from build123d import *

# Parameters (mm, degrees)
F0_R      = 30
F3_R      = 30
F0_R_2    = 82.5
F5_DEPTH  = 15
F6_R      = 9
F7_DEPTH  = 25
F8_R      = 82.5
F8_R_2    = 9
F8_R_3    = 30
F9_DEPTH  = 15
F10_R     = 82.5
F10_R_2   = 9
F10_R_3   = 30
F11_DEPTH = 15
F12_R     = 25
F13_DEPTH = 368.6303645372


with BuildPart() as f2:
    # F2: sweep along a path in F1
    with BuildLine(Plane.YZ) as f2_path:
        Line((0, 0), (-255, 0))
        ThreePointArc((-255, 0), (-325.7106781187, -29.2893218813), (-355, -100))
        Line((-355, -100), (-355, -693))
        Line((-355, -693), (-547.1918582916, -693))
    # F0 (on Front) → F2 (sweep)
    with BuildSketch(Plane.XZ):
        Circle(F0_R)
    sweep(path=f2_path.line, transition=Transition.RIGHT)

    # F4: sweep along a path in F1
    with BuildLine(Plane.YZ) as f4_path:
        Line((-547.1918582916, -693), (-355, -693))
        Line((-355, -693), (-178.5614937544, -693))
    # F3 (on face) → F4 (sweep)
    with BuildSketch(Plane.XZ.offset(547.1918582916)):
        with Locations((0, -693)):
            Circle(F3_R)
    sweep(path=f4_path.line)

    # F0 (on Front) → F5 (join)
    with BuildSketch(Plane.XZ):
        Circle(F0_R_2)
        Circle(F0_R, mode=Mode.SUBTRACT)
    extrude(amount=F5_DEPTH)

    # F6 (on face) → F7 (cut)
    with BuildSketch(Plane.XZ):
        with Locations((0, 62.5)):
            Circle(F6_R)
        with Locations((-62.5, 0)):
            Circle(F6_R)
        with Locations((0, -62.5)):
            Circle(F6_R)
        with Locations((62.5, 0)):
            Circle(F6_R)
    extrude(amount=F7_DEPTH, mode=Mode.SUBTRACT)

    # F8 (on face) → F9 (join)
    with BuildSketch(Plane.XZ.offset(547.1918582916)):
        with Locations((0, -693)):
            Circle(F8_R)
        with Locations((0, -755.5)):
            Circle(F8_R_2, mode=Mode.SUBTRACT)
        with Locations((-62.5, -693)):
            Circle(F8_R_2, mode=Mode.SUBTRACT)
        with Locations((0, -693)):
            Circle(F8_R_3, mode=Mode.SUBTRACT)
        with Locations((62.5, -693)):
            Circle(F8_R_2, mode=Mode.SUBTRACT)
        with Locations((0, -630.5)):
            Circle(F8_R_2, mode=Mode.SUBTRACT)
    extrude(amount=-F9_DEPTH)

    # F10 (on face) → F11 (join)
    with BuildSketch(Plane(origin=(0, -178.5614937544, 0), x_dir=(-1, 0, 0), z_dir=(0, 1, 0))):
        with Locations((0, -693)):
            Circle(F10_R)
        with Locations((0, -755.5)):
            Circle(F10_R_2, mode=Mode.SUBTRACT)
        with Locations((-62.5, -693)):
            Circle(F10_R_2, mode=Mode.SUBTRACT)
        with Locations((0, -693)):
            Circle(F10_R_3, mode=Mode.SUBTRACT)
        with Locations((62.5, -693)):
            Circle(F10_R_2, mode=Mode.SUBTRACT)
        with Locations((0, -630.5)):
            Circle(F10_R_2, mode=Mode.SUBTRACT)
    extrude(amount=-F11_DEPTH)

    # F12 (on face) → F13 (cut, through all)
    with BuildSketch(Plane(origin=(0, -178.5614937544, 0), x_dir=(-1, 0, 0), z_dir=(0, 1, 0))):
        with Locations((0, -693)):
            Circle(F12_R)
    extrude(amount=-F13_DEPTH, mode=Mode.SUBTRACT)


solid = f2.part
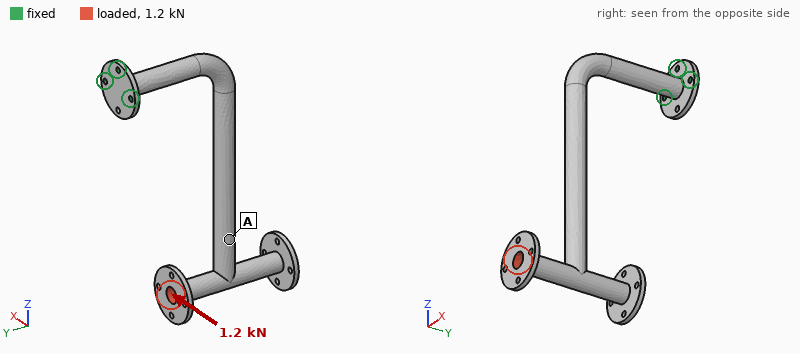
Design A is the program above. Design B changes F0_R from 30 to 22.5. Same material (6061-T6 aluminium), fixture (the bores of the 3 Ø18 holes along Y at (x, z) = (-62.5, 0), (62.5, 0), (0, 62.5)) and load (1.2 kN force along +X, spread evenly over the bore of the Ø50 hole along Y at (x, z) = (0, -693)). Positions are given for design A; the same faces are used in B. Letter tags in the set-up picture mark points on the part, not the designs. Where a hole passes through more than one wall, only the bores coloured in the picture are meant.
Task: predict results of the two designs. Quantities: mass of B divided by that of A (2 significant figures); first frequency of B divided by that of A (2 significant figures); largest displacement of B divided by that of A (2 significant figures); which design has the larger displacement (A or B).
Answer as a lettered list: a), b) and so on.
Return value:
a) 0.69
b) 0.64
c) 3.1
d) B
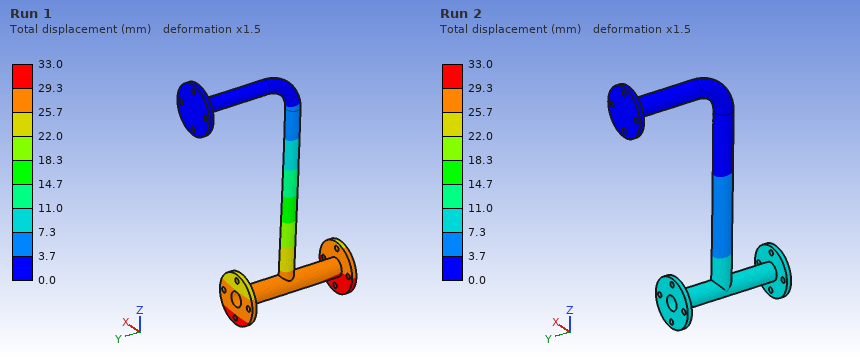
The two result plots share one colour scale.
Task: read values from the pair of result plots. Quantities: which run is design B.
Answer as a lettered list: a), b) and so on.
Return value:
a) Run 1
